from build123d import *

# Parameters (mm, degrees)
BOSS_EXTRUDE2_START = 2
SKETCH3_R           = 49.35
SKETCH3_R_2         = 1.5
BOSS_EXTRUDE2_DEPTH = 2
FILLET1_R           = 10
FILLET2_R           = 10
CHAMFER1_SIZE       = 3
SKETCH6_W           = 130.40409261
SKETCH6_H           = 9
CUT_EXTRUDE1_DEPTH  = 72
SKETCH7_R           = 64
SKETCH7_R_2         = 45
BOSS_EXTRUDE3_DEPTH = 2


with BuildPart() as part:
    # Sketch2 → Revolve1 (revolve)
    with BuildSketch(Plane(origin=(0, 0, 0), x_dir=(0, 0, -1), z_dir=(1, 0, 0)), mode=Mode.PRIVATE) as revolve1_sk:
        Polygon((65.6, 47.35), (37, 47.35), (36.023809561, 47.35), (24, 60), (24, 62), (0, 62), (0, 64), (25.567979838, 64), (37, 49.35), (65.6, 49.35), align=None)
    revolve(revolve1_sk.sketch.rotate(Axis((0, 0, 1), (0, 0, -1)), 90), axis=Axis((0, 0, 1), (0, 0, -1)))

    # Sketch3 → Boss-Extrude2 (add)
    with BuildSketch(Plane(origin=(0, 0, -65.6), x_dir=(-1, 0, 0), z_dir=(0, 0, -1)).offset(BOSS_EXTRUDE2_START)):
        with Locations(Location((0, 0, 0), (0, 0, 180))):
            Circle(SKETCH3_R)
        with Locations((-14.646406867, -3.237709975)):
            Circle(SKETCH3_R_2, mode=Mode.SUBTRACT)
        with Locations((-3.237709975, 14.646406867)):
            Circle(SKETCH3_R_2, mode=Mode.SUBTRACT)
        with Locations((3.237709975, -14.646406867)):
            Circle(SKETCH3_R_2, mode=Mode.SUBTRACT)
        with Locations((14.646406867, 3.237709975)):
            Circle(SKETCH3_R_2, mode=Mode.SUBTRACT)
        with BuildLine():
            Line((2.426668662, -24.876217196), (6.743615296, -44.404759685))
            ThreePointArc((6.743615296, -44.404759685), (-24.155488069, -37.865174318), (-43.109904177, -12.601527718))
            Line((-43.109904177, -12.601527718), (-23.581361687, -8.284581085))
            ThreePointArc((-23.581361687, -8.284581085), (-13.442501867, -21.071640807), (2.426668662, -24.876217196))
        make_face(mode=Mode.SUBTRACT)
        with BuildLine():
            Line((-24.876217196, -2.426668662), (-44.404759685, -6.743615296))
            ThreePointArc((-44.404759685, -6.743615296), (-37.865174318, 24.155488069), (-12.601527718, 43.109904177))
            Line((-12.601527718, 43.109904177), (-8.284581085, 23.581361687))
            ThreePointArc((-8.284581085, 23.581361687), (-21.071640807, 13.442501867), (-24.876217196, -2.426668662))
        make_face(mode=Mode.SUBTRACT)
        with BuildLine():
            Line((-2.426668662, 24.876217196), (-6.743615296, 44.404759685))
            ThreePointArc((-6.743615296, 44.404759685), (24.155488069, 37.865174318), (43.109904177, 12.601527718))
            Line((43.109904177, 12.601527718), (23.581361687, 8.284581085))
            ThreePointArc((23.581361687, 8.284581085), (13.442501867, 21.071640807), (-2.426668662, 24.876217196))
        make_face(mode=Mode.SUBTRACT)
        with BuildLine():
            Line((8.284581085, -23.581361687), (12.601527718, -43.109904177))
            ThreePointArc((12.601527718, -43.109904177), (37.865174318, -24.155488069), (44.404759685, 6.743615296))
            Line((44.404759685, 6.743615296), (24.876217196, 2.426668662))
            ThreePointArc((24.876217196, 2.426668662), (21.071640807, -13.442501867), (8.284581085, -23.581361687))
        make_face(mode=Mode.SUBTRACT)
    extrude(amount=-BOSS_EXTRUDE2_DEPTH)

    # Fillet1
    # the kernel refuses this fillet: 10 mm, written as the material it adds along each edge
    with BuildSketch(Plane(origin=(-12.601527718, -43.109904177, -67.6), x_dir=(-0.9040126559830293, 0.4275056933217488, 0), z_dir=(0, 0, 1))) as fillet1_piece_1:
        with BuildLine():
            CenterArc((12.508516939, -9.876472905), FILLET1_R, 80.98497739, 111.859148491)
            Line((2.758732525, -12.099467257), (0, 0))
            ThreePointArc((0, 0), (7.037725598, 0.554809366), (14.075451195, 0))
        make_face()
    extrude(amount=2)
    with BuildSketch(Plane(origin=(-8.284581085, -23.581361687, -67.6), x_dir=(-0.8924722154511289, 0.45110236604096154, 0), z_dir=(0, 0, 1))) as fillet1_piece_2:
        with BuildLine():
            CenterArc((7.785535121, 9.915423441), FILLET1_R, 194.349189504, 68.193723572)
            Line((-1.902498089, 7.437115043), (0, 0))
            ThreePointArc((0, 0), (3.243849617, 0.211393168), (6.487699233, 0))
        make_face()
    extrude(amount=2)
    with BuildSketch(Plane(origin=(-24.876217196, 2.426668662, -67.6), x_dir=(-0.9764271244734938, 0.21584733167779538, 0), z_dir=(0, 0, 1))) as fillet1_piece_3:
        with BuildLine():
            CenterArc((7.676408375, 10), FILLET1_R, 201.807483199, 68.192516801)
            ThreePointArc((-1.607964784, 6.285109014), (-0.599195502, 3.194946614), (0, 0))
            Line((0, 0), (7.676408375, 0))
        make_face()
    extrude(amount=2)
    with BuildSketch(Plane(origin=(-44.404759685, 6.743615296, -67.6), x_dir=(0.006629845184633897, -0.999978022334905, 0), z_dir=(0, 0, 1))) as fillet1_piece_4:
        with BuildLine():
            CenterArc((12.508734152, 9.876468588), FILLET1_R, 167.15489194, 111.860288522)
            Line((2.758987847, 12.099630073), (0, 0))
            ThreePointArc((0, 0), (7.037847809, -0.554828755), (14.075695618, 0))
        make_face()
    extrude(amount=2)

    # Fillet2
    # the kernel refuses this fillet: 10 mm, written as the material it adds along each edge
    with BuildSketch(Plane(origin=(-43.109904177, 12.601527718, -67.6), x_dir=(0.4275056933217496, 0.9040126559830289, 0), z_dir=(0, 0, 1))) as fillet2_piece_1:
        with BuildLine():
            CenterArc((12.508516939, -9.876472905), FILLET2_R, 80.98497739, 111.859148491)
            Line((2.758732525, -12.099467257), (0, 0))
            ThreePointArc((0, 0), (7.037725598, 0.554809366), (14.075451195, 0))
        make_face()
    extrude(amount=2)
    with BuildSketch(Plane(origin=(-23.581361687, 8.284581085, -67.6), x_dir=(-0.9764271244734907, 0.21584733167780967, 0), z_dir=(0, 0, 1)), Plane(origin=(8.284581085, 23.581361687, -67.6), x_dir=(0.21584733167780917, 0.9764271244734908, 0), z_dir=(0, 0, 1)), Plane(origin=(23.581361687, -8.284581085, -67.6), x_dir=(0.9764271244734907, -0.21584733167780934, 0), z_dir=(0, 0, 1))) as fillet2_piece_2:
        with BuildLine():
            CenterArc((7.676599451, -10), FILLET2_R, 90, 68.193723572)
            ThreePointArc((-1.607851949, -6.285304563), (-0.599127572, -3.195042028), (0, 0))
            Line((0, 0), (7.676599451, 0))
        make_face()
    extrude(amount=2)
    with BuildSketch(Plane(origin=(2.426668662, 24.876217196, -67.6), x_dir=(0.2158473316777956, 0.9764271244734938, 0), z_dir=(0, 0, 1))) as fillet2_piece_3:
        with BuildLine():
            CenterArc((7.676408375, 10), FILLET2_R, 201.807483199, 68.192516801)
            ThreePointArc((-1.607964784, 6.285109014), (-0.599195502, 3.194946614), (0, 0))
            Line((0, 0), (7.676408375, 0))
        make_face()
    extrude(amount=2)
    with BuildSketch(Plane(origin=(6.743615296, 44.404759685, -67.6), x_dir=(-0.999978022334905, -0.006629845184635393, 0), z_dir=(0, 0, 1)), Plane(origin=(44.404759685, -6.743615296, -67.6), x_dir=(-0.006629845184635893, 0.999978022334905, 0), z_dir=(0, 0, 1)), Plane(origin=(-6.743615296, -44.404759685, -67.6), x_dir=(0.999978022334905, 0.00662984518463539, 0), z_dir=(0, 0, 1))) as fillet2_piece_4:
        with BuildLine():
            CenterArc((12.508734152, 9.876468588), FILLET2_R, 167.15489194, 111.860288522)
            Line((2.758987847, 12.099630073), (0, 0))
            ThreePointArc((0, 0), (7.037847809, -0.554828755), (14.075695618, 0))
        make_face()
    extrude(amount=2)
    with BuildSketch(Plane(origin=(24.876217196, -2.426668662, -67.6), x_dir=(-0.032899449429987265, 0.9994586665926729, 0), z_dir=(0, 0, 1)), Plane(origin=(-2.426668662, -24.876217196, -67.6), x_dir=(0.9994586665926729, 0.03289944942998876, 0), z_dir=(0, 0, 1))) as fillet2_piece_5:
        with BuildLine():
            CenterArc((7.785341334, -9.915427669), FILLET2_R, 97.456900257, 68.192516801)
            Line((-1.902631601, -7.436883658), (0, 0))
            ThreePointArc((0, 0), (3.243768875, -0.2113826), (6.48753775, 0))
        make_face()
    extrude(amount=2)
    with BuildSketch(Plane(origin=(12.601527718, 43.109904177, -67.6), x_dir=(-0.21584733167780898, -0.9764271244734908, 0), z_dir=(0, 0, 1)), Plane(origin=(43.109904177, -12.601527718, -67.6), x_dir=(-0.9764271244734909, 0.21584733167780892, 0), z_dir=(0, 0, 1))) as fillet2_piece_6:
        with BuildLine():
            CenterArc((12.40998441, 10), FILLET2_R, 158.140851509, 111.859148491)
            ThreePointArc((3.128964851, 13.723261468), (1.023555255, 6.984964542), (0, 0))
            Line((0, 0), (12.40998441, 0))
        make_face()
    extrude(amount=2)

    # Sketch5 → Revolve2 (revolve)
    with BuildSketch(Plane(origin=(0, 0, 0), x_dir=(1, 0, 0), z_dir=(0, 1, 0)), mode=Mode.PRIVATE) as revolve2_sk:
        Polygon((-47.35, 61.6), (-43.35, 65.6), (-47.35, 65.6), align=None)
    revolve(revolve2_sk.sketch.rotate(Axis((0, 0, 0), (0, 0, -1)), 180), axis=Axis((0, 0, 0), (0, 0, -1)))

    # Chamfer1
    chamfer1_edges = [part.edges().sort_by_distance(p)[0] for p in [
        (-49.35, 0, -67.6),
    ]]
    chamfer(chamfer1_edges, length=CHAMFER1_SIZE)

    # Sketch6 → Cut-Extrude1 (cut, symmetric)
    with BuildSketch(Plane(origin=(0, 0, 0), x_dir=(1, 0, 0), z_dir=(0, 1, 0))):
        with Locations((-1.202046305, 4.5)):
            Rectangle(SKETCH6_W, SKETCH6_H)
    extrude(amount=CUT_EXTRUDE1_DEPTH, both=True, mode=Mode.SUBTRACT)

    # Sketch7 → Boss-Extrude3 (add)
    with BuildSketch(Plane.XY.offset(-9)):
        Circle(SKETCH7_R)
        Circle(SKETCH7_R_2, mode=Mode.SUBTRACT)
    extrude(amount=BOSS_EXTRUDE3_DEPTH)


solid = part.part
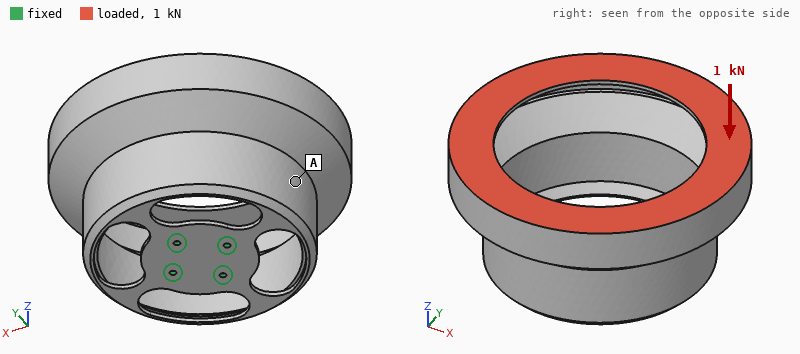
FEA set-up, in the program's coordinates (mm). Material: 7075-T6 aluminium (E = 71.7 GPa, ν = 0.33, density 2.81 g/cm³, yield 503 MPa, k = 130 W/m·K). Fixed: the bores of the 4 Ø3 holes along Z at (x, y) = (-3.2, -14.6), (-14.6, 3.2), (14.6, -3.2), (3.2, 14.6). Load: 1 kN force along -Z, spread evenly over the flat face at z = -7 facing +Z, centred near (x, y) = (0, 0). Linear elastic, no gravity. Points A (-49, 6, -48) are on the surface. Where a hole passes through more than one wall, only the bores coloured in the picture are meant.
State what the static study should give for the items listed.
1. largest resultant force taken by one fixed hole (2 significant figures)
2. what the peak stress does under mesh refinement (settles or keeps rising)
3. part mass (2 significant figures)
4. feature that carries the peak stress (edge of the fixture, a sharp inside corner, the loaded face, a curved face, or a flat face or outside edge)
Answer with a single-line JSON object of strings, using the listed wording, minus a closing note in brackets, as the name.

{"largest resultant force taken by one fixed hole": "290 N", "what the peak stress does under mesh refinement": "keeps rising", "part mass": "200 g", "feature that carries the peak stress": "edge of the fixture"}
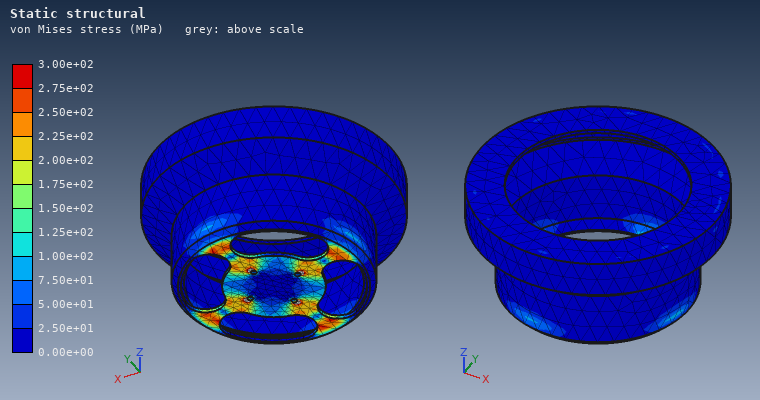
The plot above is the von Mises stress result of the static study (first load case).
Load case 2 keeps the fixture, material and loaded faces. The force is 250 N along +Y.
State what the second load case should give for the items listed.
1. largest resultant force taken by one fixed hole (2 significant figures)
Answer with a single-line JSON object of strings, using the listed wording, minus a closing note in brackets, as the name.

{"largest resultant force taken by one fixed hole": "300 N"}
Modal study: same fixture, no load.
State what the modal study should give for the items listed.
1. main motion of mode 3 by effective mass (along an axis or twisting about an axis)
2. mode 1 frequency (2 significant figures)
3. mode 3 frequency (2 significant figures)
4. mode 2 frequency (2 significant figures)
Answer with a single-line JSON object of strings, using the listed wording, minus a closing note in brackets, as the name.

{"main motion of mode 3 by effective mass": "along Z", "mode 1 frequency": "170 Hz", "mode 3 frequency": "410 Hz", "mode 2 frequency": "170 Hz"}
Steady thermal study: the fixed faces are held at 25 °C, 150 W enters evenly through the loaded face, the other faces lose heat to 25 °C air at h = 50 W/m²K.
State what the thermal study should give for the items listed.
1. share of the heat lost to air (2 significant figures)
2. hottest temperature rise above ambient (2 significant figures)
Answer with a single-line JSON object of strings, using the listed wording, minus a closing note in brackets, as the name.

{"share of the heat lost to air": "93 %", "hottest temperature rise above ambient": "81 K"}
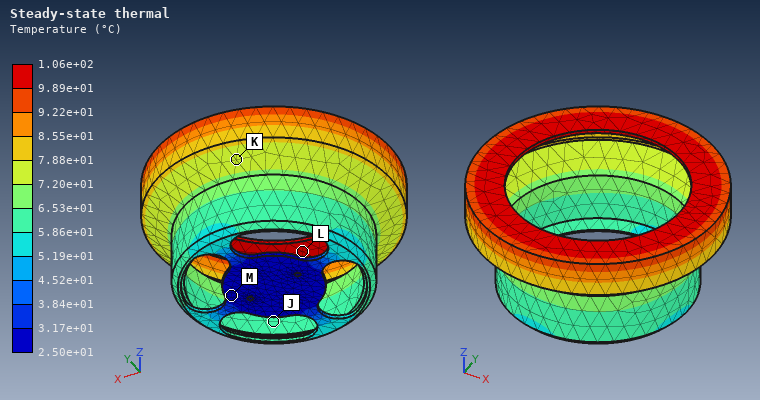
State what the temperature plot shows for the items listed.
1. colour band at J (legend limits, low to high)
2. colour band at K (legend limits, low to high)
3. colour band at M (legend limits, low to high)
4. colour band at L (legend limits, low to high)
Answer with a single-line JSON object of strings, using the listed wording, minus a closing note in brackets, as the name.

{"colour band at J": "5.86e+01 to 6.53e+01 °C", "colour band at K": "7.20e+01 to 7.88e+01 °C", "colour band at M": "2.50e+01 to 3.17e+01 °C", "colour band at L": "9.89e+01 to 1.06e+02 °C"}
